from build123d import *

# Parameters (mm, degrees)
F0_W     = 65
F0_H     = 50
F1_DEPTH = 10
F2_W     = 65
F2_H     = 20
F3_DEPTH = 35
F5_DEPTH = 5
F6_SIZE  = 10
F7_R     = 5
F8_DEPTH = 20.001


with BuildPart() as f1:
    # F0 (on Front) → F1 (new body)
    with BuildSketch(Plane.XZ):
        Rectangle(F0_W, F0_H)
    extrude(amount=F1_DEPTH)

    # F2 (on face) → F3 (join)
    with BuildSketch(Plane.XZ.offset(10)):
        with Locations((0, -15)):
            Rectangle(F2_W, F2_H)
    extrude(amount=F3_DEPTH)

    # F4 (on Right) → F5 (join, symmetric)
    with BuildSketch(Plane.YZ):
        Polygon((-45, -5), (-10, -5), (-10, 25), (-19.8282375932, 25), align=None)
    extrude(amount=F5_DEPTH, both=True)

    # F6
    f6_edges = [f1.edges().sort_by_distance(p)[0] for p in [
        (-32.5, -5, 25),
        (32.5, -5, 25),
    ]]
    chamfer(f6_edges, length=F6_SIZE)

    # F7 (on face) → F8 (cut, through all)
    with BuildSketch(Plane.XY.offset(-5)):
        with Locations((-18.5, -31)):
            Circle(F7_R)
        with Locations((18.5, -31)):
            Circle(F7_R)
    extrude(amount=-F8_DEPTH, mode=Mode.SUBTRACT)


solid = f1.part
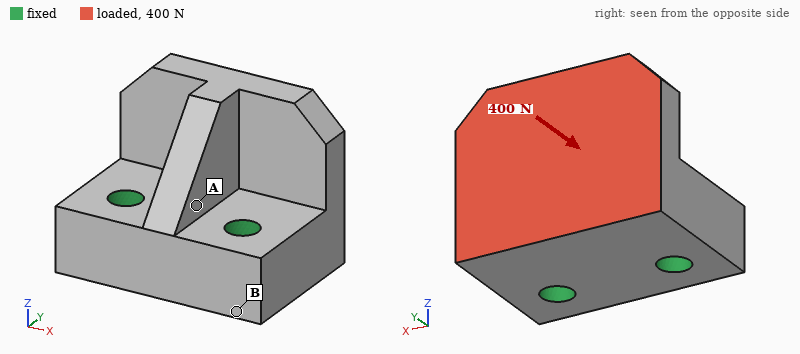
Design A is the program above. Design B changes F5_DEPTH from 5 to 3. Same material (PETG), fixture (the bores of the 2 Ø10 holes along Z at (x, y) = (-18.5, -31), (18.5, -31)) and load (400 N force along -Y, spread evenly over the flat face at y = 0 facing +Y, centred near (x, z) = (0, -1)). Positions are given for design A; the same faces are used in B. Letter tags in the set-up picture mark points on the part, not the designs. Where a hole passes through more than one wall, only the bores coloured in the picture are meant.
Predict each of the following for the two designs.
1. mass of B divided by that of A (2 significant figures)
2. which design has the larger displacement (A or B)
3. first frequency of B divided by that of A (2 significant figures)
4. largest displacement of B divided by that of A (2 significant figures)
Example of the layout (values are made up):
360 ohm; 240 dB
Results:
0.97; B; 0.99; 1.1
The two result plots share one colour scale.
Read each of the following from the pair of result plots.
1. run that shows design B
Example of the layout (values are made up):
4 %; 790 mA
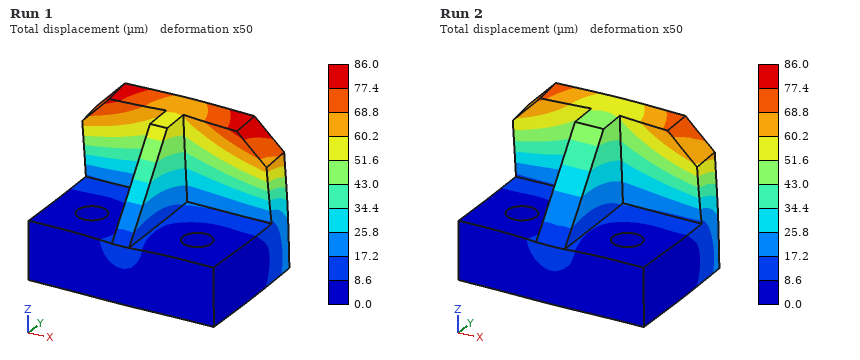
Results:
Run 1
